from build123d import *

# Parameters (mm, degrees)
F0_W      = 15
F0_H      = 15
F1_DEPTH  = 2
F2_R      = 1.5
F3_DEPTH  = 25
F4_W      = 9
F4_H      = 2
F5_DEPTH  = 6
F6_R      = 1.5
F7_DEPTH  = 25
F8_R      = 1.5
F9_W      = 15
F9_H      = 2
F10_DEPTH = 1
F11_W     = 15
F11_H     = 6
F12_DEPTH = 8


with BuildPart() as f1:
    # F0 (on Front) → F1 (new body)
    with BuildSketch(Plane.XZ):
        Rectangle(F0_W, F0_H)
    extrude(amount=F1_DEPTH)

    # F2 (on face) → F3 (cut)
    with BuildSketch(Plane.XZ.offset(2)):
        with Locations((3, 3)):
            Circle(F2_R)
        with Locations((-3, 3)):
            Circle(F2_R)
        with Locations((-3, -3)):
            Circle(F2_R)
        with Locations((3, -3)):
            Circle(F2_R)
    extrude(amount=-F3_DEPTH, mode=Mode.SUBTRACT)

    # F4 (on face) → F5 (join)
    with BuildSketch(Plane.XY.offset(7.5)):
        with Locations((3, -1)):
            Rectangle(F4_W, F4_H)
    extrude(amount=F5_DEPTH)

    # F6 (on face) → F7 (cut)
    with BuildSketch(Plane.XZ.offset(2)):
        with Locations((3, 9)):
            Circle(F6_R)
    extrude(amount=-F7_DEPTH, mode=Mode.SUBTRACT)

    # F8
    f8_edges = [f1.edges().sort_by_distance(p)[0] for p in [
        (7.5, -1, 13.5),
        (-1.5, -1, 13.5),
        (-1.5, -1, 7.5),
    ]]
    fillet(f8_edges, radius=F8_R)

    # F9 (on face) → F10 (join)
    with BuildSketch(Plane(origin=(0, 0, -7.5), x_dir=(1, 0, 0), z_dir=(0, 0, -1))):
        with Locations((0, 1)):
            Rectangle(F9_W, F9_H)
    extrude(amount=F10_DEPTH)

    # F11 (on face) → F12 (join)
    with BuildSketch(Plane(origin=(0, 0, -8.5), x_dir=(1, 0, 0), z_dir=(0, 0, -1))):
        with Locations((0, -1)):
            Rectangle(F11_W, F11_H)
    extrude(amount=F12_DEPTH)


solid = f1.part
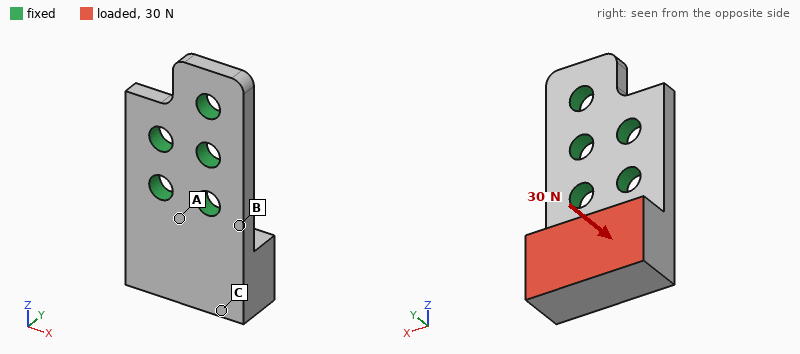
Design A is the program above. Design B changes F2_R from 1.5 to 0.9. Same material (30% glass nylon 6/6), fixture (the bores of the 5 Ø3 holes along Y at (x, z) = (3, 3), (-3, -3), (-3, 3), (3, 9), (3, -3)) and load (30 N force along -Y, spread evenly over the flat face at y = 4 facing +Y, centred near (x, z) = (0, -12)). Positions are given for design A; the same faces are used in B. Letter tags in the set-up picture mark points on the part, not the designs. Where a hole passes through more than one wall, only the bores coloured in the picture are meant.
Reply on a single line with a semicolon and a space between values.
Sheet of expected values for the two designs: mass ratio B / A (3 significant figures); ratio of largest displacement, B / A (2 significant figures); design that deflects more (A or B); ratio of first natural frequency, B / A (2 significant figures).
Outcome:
1.03; 1.3; B; 0.89
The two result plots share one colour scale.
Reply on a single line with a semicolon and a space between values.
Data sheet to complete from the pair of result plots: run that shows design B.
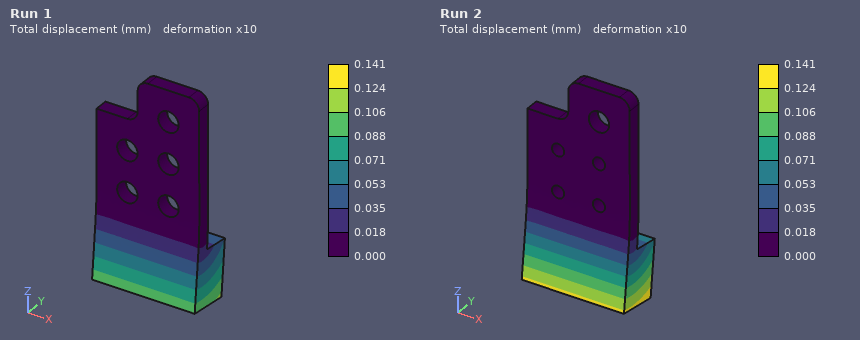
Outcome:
Run 2
